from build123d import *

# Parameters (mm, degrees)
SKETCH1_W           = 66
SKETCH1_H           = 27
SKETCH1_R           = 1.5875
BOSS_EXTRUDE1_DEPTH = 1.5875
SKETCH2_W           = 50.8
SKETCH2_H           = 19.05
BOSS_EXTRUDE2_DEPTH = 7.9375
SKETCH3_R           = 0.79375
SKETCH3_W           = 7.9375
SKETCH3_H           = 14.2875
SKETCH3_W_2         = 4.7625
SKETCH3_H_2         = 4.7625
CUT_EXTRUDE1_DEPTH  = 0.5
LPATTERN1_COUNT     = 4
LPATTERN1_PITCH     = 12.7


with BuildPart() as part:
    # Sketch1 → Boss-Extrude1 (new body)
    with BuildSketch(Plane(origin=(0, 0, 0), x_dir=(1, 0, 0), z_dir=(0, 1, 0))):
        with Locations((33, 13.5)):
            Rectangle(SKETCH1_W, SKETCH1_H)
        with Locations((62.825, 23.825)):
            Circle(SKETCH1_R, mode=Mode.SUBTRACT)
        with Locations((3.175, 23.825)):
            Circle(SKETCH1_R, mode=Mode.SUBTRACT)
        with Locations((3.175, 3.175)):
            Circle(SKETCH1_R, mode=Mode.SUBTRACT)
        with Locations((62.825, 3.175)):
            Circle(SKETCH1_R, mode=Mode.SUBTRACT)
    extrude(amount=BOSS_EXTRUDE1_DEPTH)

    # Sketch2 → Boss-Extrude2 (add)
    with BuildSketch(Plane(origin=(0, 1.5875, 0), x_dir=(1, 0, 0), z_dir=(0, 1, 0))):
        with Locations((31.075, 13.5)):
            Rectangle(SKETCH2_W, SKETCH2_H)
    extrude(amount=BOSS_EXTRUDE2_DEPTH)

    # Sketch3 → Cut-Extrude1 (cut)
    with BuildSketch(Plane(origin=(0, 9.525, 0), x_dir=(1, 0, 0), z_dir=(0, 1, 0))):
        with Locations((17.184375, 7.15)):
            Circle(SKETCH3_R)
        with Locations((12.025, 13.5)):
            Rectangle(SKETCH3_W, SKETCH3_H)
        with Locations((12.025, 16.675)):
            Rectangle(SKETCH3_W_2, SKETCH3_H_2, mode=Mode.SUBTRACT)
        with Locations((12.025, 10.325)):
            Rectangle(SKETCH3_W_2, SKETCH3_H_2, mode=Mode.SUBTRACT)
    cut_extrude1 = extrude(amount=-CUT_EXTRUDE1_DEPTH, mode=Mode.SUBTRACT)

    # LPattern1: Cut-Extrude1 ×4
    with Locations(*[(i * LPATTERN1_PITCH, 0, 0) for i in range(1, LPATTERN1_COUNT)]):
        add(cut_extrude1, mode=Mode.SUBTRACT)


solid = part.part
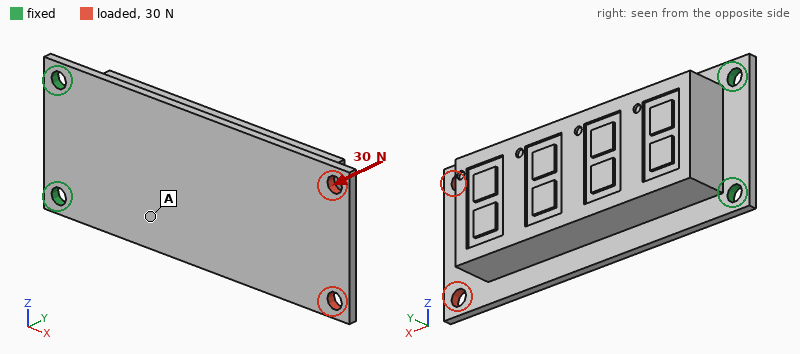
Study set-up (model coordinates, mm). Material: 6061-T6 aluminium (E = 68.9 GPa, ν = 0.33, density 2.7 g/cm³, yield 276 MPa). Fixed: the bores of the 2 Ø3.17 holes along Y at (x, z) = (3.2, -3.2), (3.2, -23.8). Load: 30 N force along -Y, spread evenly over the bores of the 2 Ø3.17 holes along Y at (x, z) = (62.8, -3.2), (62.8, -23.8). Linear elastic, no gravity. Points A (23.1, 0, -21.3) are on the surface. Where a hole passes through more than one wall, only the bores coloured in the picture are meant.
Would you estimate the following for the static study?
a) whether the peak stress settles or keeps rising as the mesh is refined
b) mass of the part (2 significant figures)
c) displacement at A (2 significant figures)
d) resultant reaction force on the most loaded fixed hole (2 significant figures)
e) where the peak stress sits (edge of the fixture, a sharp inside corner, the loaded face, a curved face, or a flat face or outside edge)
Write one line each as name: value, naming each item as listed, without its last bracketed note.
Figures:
whether the peak stress settles or keeps rising as the mesh is refined: keeps rising
mass of the part: 28 g
displacement at A: 0.17 mm
resultant reaction force on the most loaded fixed hole: 17 N
where the peak stress sits: edge of the fixture
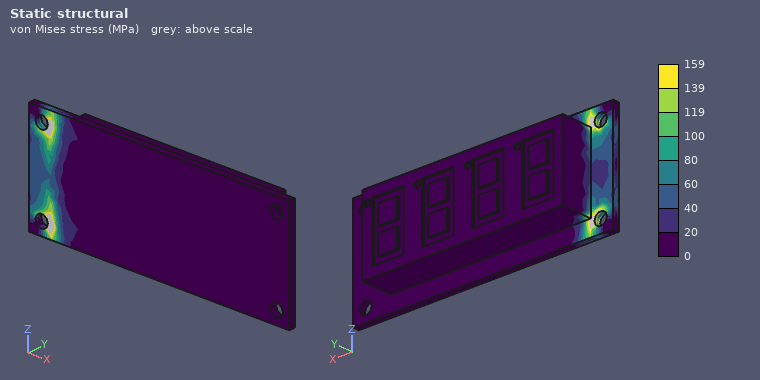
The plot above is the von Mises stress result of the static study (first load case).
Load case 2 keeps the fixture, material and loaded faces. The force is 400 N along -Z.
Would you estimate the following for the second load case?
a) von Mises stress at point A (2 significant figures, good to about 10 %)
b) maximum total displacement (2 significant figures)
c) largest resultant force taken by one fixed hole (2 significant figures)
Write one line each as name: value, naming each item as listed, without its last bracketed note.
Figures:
von Mises stress at point A: 22 MPa
maximum total displacement: 0.13 mm
largest resultant force taken by one fixed hole: 1.1 kN
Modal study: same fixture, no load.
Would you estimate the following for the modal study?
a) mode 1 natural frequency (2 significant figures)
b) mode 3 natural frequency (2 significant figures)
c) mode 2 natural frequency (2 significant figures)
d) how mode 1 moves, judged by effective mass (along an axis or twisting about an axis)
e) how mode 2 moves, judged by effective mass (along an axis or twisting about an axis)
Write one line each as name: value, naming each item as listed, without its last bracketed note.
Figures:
mode 1 natural frequency: 410 Hz
mode 3 natural frequency: 7000 Hz
mode 2 natural frequency: 3800 Hz
how mode 1 moves, judged by effective mass: along Y
how mode 2 moves, judged by effective mass: along Z
